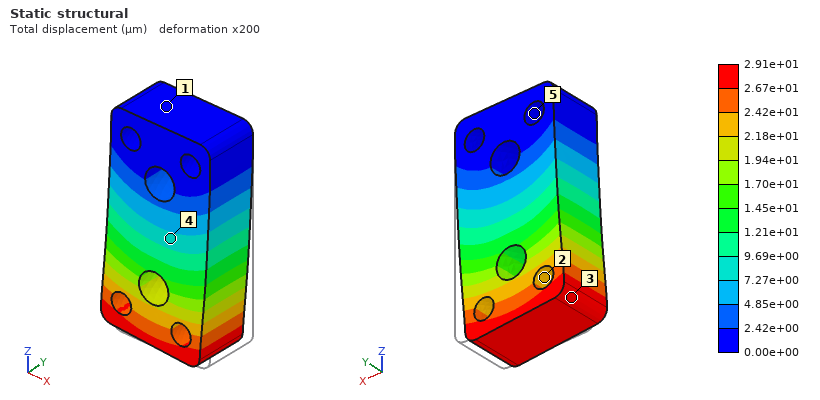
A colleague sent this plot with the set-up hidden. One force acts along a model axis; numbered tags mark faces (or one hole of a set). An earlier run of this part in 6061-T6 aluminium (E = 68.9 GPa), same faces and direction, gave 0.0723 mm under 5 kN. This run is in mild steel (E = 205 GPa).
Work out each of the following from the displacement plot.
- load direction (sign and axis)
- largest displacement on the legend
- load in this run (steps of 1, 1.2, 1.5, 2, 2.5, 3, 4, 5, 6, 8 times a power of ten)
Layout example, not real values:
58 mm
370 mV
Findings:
-X
2.91e+01 µm
6 kN
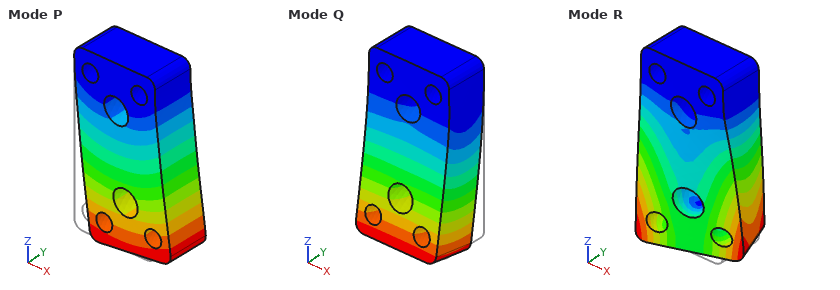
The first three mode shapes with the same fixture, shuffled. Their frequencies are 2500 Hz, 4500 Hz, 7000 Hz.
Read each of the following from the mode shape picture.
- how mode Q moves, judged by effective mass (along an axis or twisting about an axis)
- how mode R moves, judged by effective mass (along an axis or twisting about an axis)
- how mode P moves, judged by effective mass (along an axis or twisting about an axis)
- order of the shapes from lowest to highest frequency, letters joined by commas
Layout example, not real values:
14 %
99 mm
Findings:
along Y
twisting about Z
along X
Q, P, R
